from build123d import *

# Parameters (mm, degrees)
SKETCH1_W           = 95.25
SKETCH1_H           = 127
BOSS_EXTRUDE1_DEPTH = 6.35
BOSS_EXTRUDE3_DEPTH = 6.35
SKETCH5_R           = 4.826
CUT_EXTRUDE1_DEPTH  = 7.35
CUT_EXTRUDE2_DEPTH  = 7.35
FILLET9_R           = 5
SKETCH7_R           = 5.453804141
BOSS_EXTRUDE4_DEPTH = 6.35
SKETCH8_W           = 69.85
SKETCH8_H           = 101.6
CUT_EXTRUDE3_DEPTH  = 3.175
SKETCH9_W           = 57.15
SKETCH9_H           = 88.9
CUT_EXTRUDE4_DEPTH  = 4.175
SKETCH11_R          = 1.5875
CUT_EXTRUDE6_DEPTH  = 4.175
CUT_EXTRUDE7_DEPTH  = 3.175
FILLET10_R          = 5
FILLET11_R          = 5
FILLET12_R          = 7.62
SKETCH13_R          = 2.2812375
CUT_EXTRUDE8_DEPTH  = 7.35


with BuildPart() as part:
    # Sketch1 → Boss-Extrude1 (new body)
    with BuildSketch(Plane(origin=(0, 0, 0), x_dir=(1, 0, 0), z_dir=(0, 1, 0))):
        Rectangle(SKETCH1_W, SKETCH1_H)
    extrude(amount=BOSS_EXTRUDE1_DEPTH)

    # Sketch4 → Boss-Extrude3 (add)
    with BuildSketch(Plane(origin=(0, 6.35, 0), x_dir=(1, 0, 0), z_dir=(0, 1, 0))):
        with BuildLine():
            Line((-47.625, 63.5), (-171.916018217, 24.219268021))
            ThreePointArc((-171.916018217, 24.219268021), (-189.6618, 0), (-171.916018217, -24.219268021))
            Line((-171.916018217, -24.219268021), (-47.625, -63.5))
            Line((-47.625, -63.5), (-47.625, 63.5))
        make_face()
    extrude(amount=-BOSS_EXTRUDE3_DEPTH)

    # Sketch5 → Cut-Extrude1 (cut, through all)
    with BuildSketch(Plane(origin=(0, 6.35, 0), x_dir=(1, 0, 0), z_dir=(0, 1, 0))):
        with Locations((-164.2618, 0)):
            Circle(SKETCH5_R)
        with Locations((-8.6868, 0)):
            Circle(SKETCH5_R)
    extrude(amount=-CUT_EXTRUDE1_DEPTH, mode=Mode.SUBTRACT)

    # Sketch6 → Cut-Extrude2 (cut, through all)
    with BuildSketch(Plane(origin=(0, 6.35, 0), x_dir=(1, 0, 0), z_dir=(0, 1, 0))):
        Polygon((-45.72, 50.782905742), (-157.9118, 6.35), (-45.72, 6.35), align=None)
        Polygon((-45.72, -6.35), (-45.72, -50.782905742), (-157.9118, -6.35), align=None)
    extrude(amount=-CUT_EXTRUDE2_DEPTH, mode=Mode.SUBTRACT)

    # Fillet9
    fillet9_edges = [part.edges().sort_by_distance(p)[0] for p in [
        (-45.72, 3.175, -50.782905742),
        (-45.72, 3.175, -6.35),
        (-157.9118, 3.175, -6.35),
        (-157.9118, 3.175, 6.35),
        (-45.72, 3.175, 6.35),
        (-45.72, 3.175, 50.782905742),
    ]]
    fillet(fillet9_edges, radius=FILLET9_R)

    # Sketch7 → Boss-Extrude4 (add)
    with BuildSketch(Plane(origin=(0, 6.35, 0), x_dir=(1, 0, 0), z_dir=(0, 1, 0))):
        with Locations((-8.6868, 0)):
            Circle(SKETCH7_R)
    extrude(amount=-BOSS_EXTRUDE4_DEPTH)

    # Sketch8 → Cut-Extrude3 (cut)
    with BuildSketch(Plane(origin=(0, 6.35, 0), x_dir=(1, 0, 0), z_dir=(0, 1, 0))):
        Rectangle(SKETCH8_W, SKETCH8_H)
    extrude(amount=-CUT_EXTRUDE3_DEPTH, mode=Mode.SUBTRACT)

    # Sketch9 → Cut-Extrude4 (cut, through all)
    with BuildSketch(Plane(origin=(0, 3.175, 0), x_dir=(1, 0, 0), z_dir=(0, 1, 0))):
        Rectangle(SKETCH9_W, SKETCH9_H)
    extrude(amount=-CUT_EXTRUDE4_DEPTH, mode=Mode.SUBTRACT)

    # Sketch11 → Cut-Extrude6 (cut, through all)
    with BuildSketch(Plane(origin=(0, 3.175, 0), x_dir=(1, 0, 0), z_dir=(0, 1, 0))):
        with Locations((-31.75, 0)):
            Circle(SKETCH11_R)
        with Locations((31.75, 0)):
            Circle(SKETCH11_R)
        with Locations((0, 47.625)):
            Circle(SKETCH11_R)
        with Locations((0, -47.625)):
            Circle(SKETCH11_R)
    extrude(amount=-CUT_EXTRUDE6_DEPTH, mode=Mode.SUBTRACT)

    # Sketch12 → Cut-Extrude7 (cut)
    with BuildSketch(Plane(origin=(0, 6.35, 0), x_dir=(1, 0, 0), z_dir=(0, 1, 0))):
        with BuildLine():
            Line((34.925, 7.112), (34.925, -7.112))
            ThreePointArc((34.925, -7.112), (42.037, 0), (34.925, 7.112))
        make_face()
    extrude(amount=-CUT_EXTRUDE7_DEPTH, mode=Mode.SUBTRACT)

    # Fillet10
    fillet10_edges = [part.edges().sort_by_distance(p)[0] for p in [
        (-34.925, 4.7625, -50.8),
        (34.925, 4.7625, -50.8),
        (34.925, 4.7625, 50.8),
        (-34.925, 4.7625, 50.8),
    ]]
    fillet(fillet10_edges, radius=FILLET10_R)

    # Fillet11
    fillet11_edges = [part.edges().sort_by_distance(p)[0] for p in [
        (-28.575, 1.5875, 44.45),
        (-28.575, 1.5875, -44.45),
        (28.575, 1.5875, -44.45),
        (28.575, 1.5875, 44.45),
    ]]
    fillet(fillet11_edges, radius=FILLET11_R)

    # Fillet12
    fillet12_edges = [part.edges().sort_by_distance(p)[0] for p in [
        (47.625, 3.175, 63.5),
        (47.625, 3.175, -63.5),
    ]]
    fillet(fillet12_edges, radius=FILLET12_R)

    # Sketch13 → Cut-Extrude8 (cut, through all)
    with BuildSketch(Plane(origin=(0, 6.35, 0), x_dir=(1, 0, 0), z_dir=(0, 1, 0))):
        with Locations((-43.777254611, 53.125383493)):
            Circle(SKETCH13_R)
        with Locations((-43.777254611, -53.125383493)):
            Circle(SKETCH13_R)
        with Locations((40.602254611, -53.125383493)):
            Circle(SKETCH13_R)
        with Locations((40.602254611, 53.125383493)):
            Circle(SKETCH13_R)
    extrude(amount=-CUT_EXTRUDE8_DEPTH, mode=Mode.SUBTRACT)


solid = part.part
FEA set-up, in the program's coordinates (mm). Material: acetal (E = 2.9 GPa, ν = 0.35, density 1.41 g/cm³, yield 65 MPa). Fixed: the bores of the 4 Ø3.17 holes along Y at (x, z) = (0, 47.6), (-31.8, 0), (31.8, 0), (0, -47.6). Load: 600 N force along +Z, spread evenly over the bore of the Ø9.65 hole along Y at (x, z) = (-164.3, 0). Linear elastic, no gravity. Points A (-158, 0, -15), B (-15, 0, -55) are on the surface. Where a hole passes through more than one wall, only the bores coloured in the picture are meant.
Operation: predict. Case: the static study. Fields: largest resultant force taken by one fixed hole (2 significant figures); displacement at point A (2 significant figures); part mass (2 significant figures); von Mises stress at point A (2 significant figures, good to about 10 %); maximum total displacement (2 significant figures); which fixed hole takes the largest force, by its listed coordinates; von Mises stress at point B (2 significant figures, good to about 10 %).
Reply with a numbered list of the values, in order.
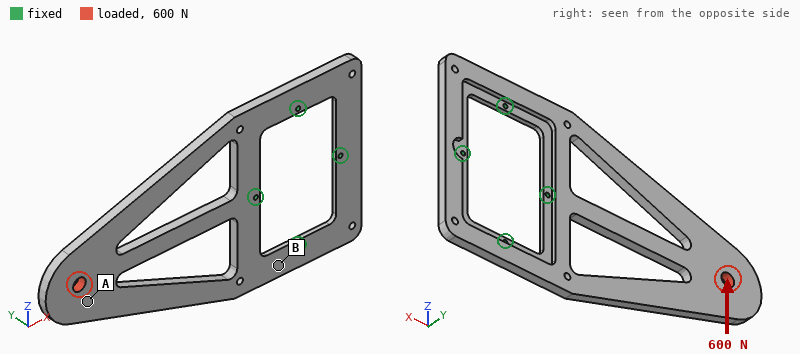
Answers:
1. 800 N
2. 1.6 mm
3. 110 g
4. 3.3 MPa
5. 1.6 mm
6. (-31.8, 0)
7. 7.6 MPa
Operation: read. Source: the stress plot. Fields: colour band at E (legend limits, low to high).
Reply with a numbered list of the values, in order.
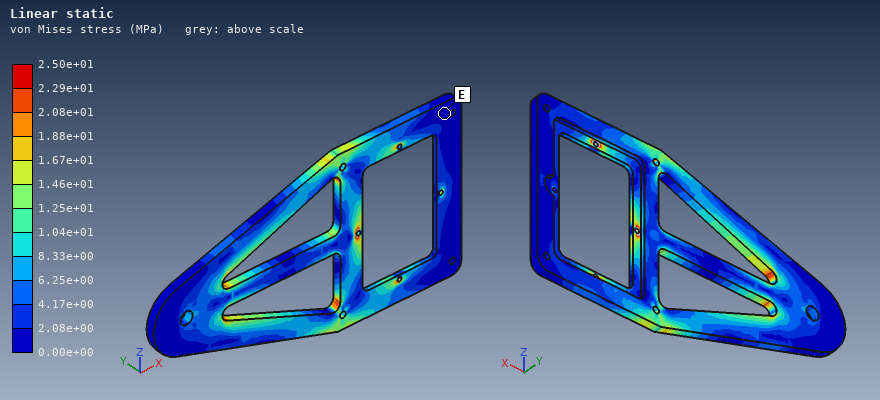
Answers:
1. 0.00e+00 to 2.08e+00 MPa
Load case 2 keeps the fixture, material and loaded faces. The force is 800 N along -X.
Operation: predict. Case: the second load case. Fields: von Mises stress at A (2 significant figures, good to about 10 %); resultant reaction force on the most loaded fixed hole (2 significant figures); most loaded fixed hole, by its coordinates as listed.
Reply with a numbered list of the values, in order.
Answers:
1. 2.0 MPa
2. 310 N
3. (-31.8, 0)
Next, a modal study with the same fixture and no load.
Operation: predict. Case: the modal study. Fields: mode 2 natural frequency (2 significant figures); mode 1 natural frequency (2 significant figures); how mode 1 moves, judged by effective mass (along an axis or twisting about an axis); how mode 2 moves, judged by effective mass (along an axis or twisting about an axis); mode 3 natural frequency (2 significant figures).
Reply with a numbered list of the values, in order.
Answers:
1. 180 Hz
2. 43 Hz
3. along Y
4. twisting about X
5. 270 Hz
